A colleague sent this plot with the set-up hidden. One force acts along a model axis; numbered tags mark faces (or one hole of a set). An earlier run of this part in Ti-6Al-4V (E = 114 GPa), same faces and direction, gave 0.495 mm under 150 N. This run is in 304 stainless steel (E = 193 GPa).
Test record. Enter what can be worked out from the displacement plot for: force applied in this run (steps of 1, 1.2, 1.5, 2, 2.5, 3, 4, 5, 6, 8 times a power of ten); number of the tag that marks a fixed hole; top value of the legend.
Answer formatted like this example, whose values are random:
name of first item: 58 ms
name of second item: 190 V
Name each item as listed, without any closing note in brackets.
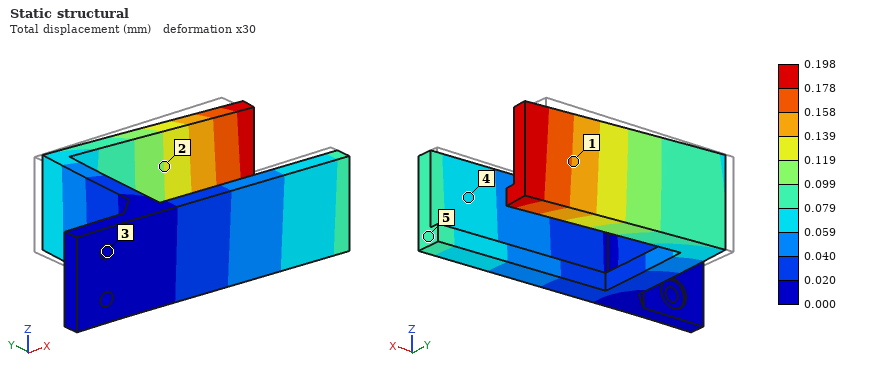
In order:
force applied in this run: 100 N
number of the tag that marks a fixed hole: 3
top value of the legend: 0.198 mm
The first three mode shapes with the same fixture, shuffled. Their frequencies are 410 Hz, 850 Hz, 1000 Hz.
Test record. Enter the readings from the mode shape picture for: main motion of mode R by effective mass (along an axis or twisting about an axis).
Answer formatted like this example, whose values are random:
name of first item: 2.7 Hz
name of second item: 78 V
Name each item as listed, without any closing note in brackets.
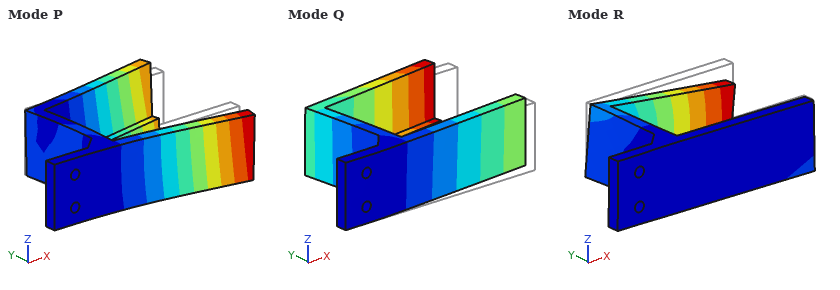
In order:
main motion of mode R by effective mass: along Z
